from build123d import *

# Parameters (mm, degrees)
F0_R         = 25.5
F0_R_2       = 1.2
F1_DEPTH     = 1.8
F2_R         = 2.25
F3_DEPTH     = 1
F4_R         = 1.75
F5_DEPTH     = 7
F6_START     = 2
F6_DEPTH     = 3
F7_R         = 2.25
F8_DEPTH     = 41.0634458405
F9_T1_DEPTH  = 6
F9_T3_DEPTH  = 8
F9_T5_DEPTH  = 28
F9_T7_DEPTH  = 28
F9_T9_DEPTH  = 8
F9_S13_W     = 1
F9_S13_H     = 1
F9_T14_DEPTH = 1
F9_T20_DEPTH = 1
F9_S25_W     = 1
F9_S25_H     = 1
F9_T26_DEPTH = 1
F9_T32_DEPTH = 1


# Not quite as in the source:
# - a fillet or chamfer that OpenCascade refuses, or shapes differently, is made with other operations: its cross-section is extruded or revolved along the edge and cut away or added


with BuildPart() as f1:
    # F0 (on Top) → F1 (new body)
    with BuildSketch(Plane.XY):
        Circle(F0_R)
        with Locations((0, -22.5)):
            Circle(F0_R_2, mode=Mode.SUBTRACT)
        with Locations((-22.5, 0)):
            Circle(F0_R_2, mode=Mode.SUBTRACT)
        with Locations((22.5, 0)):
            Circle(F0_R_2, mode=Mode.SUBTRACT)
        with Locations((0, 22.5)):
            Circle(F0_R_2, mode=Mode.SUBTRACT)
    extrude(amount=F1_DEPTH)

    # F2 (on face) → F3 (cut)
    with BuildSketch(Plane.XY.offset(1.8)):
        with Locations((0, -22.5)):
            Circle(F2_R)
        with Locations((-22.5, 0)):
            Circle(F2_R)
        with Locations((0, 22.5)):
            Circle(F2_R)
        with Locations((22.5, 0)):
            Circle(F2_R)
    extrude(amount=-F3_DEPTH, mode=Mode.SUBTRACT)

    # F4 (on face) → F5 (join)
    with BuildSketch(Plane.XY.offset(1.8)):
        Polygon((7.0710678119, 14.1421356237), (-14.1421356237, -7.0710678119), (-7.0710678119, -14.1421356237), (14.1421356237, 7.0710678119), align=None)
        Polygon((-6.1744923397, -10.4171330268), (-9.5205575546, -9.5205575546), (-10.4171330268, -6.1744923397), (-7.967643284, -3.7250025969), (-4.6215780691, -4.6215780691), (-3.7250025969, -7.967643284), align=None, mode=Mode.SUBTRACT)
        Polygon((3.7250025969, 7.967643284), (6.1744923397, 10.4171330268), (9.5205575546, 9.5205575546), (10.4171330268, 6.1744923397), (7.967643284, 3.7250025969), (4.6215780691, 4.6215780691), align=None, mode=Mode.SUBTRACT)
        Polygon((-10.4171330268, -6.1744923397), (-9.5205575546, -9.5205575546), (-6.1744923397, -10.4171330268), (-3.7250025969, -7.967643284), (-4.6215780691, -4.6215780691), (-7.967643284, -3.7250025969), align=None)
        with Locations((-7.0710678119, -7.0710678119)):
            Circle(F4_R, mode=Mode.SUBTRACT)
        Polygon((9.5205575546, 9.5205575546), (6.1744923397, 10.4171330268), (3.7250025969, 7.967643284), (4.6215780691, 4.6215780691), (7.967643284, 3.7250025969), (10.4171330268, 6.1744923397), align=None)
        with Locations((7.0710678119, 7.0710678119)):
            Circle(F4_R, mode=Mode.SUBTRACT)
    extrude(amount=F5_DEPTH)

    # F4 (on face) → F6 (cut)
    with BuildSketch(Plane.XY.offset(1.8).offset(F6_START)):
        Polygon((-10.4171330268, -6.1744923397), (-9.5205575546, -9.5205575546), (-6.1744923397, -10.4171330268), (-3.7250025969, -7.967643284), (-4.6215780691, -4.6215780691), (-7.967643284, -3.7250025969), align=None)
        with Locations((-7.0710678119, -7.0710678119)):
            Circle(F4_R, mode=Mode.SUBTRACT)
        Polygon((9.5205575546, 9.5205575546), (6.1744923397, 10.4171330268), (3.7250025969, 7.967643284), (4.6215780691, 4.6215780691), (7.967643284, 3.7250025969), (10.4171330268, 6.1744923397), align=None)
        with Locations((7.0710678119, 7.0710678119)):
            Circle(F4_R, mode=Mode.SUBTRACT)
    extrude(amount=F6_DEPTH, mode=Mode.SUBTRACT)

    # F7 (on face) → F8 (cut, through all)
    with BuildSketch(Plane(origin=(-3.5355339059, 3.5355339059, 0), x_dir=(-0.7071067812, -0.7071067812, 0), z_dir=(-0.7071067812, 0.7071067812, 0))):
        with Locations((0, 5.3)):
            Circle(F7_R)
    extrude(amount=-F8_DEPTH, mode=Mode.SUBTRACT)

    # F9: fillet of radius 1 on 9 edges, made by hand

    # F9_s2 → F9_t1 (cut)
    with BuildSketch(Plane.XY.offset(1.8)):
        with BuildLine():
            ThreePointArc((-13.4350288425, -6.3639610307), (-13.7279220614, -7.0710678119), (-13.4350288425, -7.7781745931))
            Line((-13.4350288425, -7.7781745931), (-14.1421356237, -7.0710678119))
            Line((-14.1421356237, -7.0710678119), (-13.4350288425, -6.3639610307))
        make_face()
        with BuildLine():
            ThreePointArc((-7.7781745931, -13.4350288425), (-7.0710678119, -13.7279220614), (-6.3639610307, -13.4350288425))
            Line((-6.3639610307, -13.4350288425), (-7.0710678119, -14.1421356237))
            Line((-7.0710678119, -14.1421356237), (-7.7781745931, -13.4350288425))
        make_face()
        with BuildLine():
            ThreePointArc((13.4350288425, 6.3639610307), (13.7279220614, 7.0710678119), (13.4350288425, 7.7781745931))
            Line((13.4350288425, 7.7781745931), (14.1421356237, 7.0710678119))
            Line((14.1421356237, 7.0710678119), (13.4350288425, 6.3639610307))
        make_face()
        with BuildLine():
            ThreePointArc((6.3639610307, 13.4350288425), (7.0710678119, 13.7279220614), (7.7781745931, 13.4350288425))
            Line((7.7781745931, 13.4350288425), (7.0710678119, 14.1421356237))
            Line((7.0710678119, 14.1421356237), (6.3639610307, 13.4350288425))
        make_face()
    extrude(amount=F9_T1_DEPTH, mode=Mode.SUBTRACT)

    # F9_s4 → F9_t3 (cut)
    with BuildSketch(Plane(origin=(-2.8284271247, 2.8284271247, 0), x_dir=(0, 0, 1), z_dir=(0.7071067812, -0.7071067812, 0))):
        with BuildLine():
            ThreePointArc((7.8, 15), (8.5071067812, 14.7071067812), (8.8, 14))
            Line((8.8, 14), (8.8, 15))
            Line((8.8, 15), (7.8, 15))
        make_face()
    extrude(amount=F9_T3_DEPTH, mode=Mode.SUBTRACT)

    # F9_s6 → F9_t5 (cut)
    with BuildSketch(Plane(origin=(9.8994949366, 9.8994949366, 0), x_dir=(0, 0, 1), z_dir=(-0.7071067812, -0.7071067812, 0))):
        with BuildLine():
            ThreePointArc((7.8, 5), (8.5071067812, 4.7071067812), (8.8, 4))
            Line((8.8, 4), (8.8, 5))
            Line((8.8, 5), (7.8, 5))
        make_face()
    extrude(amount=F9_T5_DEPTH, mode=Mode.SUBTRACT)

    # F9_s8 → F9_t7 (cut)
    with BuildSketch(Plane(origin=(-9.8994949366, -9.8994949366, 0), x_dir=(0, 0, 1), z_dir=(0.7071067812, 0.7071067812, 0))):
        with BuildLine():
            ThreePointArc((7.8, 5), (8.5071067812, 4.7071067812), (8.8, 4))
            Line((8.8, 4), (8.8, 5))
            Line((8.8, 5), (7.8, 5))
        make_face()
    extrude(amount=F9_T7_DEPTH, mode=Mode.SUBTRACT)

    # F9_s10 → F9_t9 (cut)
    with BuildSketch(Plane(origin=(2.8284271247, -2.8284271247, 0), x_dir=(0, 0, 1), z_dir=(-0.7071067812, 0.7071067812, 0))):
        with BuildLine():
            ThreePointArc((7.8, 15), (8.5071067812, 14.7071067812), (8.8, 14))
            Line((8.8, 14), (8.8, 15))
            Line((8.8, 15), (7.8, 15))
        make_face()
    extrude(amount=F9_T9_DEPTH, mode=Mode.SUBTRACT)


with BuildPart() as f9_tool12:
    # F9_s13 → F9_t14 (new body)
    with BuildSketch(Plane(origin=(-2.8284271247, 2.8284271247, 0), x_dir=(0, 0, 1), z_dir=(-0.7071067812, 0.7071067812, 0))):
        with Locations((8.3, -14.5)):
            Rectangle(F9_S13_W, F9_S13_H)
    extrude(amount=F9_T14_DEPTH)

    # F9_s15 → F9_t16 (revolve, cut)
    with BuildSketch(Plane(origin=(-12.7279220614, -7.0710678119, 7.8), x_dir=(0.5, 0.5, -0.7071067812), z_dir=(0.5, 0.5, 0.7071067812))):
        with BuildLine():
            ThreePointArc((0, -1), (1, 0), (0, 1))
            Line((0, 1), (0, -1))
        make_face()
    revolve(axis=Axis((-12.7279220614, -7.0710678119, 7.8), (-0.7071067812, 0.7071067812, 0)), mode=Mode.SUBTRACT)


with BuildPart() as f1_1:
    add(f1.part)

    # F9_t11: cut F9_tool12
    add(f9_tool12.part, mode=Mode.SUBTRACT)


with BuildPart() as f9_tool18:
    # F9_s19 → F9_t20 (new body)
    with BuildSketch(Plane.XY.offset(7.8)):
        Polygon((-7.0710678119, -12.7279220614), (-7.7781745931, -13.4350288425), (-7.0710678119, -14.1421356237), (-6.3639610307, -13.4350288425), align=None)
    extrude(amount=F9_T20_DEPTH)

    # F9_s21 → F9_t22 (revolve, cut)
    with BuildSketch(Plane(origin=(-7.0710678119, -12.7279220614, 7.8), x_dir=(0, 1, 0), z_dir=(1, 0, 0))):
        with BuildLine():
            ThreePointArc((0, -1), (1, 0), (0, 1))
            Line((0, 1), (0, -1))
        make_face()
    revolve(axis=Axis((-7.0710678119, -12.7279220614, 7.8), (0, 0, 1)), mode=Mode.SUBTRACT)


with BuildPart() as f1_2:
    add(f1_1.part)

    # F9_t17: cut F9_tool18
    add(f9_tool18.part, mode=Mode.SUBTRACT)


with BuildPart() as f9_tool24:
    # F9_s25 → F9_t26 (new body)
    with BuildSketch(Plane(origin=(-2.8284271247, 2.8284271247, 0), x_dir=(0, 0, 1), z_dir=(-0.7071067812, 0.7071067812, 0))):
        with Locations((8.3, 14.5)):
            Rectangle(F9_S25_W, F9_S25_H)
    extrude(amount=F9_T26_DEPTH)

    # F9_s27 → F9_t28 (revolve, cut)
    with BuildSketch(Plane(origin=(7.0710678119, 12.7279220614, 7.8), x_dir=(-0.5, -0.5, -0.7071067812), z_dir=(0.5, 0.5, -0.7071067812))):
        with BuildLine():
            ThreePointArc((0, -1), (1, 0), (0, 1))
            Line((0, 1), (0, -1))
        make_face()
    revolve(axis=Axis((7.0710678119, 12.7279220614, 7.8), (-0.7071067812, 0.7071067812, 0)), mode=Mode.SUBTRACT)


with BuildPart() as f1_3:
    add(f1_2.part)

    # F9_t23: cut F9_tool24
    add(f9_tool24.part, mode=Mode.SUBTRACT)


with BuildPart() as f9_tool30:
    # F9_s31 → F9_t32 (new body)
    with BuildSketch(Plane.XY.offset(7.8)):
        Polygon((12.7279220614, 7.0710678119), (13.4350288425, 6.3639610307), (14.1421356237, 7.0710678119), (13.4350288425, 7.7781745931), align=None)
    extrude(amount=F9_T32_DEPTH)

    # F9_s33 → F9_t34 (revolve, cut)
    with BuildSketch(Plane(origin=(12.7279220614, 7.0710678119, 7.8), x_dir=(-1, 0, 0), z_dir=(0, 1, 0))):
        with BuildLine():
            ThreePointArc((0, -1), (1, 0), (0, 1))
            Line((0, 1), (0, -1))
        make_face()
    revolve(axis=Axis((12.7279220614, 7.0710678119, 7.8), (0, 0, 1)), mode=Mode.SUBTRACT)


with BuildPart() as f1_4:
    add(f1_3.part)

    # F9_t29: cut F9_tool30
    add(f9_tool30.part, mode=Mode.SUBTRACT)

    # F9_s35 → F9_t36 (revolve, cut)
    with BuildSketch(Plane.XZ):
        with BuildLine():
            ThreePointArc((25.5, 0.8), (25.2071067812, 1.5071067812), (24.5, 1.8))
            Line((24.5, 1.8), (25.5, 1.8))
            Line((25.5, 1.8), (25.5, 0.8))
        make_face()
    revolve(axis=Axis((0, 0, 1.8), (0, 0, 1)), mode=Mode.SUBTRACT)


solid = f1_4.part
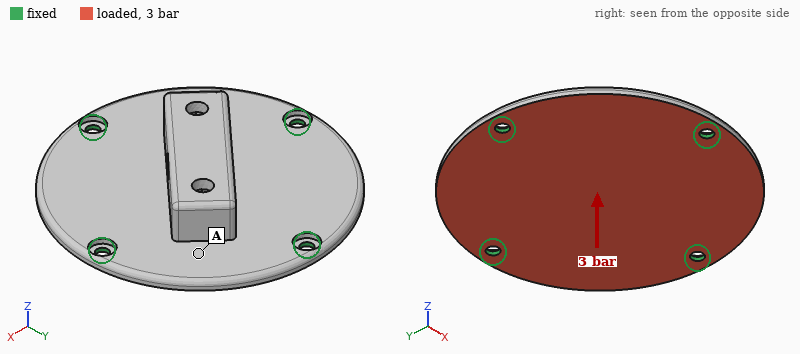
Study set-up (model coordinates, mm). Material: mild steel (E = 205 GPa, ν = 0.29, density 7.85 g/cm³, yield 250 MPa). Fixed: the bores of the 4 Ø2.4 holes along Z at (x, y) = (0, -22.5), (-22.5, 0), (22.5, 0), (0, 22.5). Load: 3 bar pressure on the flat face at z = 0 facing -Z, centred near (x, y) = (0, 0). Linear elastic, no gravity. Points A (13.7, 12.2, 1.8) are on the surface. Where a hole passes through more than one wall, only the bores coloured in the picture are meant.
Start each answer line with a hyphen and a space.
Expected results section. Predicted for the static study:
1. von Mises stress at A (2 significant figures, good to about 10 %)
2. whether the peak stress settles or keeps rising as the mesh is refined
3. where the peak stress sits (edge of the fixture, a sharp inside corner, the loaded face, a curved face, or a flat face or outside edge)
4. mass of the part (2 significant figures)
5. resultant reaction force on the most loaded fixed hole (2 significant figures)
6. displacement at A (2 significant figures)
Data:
- 23 MPa
- keeps rising
- edge of the fixture
- 41 g
- 240 N
- 14 µm
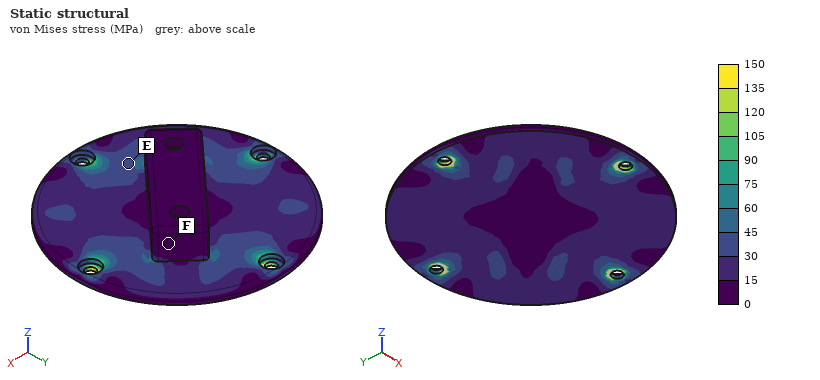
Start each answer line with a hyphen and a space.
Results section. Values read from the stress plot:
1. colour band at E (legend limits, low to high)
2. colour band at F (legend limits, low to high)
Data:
- 30 to 45 MPa
- 0 to 15 MPa
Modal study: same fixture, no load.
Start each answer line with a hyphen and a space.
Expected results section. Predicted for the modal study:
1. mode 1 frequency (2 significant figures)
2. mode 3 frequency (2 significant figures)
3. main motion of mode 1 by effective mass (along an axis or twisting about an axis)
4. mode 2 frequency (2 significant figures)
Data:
- 4800 Hz
- 7100 Hz
- along Z
- 6300 Hz
